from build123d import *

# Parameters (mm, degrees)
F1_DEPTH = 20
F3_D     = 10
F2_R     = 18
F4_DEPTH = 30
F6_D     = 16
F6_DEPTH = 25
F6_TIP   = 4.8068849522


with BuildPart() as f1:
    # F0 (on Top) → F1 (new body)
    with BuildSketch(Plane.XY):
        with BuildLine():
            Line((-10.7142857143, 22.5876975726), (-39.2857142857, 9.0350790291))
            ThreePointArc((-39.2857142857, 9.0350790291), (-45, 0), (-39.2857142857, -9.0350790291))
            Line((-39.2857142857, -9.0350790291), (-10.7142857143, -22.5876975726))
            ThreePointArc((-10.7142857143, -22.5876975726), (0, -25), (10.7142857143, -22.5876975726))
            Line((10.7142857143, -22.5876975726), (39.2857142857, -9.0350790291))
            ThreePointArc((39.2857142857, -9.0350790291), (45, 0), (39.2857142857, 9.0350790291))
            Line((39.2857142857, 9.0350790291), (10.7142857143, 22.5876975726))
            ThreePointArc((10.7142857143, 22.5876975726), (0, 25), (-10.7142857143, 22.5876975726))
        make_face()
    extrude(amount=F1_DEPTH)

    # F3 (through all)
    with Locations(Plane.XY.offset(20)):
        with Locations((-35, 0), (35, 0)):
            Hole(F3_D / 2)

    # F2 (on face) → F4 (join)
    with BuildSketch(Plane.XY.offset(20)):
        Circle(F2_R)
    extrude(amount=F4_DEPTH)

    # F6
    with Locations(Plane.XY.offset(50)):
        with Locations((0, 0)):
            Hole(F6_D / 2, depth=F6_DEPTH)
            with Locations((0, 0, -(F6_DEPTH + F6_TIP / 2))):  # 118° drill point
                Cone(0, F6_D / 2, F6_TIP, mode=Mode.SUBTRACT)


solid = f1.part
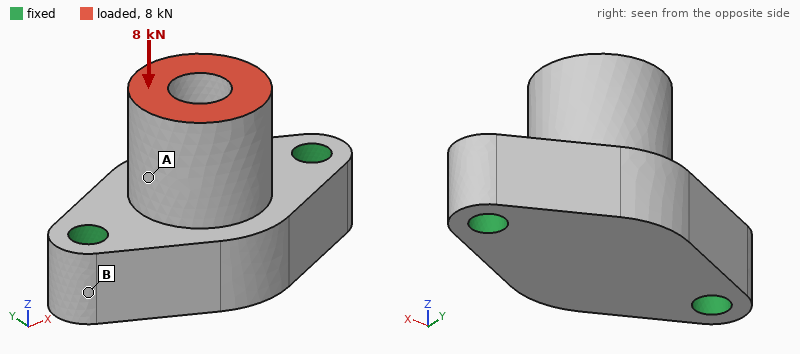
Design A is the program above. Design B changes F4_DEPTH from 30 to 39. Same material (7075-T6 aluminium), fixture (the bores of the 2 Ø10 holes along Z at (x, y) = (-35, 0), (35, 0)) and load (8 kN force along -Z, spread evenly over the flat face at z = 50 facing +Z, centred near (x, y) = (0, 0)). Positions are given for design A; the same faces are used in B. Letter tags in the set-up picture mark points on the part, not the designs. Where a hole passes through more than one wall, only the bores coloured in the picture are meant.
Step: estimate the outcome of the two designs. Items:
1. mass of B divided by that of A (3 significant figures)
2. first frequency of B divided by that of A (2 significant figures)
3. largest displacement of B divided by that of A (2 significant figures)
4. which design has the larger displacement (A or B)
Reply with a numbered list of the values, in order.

1. 1.09
2. 0.78
3. 1.1
4. B
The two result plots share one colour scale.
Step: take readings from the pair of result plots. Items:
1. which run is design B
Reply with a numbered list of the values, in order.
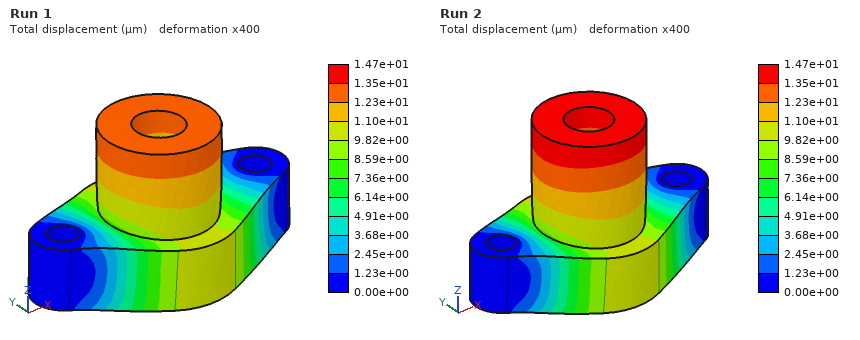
1. Run 2
